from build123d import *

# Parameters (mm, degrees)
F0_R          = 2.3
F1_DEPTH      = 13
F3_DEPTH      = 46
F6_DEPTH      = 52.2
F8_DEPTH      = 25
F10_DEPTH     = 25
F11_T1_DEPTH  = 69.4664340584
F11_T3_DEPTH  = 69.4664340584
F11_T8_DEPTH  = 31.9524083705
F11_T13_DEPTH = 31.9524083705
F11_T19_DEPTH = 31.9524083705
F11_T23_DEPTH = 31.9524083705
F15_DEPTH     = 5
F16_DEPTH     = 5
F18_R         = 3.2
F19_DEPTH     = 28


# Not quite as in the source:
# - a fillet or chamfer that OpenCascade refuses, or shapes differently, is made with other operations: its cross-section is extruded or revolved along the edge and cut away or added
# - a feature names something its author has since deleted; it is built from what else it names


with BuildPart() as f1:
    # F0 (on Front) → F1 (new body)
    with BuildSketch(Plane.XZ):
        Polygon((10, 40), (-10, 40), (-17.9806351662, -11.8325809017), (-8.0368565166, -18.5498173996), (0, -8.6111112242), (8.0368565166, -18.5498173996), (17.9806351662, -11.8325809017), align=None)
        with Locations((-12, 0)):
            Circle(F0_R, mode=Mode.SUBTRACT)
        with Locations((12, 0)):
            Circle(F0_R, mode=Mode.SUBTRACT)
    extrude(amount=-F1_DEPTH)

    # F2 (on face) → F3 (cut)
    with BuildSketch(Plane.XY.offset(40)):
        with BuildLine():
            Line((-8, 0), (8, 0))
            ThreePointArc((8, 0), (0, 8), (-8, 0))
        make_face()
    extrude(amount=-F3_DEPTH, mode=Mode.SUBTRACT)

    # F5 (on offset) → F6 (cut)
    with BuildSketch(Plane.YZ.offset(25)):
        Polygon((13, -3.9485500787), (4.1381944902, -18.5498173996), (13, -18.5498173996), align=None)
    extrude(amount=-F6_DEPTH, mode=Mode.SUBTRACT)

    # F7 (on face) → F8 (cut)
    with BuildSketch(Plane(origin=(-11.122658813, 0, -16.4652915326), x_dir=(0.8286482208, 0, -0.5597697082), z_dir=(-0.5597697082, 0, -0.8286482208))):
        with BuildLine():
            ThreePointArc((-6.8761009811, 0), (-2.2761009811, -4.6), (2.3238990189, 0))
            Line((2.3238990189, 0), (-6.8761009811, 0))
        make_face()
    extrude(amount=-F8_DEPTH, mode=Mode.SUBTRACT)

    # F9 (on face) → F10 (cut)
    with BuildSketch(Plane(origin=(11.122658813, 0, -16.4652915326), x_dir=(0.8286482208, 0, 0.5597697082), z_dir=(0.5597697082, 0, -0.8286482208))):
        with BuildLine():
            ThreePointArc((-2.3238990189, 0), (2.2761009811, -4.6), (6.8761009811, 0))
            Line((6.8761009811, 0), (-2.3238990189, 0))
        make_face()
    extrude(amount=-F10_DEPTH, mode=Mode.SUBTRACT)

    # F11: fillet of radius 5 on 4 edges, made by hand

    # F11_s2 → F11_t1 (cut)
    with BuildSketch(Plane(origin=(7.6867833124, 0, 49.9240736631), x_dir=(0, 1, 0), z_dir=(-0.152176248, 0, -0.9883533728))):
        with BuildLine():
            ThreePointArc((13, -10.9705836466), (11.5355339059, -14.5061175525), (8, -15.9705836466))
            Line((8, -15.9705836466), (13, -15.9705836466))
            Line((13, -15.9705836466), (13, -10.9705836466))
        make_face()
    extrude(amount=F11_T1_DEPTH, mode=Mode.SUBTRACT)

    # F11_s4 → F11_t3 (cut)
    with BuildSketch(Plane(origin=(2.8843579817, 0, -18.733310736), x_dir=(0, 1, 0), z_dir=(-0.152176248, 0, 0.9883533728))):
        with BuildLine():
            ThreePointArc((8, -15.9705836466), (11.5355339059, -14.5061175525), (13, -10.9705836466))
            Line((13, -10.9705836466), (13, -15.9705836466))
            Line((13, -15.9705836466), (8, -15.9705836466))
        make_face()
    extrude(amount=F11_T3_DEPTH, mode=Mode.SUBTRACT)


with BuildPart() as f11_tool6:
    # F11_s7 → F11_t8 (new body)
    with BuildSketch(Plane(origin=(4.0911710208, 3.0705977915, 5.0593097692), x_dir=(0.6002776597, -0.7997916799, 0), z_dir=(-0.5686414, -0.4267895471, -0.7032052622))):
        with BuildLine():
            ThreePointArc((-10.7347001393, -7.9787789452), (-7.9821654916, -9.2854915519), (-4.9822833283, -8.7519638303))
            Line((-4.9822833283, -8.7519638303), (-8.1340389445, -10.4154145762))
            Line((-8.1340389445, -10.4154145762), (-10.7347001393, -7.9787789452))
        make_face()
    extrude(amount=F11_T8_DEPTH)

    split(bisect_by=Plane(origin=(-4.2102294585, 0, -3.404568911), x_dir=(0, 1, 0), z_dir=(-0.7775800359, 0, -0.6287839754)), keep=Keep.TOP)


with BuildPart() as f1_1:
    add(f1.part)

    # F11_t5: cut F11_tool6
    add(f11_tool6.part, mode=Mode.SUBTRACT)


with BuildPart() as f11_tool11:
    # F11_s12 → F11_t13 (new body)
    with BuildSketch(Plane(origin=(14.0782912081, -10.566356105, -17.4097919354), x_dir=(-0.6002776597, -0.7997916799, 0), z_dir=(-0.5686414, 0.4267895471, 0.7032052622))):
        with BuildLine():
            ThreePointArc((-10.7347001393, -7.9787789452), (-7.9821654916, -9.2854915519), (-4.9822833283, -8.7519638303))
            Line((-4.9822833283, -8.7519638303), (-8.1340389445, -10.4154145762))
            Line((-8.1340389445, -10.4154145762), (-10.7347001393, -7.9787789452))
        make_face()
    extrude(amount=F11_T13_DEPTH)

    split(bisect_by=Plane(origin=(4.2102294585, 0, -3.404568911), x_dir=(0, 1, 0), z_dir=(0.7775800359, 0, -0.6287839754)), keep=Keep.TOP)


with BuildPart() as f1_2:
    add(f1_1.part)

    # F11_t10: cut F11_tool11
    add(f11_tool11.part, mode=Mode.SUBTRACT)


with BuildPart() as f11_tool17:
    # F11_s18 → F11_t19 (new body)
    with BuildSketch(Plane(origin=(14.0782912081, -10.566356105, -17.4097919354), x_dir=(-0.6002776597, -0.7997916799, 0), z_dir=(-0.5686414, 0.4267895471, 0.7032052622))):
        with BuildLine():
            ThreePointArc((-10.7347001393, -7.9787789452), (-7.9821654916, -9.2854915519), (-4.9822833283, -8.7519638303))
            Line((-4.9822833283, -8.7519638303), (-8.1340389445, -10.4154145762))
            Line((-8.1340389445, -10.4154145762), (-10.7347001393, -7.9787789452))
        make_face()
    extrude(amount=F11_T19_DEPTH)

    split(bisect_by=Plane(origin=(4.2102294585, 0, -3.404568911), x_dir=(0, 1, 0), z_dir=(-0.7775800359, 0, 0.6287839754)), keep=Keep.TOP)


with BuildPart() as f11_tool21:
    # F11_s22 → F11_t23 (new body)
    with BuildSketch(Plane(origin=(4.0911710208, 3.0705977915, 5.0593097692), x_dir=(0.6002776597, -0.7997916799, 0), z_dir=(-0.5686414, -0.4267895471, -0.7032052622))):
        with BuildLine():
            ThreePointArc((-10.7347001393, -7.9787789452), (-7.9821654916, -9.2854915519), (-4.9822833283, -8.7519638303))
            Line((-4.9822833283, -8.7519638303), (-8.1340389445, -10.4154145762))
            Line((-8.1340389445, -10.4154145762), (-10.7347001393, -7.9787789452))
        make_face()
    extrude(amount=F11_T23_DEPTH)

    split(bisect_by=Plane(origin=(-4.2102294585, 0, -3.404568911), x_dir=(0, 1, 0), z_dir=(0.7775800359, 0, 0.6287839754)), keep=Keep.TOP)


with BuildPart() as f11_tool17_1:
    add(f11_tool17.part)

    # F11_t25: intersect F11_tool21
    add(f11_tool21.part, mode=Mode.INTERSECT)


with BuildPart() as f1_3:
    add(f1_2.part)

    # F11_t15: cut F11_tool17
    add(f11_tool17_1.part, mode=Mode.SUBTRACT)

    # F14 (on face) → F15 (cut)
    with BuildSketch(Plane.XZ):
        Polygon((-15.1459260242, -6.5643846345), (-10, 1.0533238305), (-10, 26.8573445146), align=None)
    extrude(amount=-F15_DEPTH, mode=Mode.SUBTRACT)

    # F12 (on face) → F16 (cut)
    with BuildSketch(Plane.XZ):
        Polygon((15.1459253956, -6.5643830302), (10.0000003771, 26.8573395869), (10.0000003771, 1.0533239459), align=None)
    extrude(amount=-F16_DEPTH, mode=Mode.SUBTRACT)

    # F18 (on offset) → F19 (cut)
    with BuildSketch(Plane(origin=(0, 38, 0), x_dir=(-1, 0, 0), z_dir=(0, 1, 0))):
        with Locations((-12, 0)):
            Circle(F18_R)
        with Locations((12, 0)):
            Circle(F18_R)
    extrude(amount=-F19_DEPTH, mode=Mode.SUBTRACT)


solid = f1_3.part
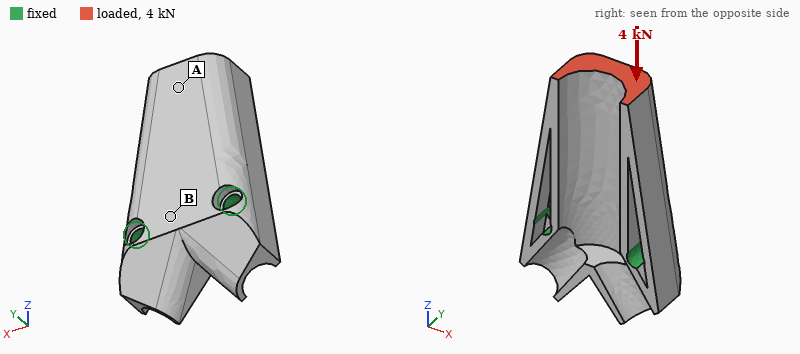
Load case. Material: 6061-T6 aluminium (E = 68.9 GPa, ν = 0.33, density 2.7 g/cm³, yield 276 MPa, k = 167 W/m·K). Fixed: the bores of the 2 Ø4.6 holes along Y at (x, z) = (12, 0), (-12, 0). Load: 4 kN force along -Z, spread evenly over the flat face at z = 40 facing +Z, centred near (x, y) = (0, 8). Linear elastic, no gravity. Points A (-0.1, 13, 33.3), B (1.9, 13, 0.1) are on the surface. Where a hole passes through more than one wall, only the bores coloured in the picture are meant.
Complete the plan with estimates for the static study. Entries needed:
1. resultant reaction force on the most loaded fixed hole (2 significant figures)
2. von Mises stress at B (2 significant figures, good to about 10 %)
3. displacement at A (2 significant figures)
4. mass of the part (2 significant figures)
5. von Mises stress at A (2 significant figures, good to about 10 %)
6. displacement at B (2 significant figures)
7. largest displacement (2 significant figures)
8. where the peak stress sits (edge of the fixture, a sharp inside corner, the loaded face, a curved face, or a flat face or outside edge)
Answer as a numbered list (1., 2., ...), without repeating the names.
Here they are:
1. 2.0 kN
2. 8.3 MPa
3. 21 µm
4. 32 g
5. 28 MPa
6. 4.5 µm
7. 25 µm
8. edge of the fixture
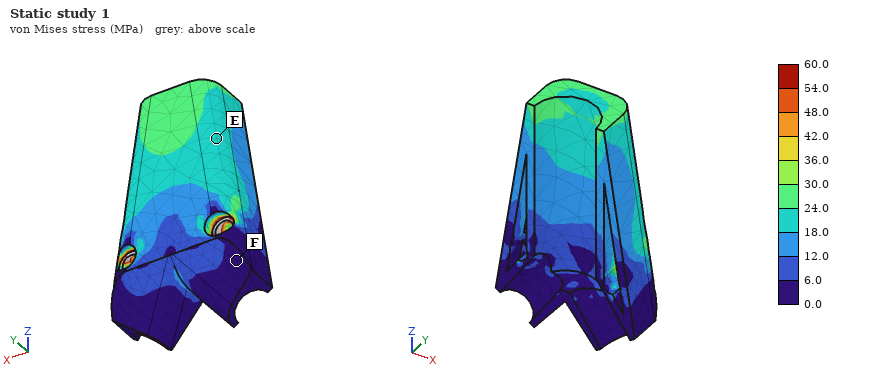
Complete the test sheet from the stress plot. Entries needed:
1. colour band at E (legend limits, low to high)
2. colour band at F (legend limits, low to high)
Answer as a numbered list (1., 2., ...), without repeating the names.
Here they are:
1. 18.0 to 24.0 MPa
2. 0.0 to 6.0 MPa
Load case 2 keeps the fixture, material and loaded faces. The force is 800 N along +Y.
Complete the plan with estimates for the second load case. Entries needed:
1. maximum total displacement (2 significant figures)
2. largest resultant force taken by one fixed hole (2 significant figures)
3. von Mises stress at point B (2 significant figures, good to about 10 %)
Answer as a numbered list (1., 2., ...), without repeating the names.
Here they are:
1. 0.14 mm
2. 430 N
3. 28 MPa
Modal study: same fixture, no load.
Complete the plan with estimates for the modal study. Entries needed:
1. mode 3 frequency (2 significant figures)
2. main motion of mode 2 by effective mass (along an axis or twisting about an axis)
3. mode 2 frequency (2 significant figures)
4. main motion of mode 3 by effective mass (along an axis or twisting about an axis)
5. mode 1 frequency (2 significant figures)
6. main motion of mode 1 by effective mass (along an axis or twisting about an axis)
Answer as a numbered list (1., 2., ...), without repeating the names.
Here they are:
1. 15 kHz
2. along X
3. 9800 Hz
4. along X
5. 5400 Hz
6. along Y
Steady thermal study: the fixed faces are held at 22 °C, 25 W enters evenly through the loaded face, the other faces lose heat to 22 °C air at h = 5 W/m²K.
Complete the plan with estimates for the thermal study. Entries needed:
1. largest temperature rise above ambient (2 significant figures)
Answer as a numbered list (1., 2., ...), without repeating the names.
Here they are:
1. 30 K
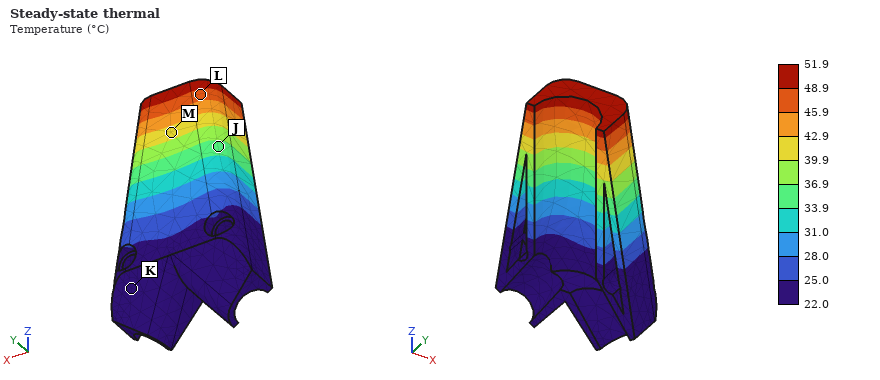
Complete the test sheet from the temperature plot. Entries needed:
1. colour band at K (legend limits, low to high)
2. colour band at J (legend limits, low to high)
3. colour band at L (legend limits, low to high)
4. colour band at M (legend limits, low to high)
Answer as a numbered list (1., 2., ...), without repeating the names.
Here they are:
1. 22.0 to 25.0 °C
2. 33.9 to 36.9 °C
3. 45.9 to 48.9 °C
4. 39.9 to 42.9 °C
